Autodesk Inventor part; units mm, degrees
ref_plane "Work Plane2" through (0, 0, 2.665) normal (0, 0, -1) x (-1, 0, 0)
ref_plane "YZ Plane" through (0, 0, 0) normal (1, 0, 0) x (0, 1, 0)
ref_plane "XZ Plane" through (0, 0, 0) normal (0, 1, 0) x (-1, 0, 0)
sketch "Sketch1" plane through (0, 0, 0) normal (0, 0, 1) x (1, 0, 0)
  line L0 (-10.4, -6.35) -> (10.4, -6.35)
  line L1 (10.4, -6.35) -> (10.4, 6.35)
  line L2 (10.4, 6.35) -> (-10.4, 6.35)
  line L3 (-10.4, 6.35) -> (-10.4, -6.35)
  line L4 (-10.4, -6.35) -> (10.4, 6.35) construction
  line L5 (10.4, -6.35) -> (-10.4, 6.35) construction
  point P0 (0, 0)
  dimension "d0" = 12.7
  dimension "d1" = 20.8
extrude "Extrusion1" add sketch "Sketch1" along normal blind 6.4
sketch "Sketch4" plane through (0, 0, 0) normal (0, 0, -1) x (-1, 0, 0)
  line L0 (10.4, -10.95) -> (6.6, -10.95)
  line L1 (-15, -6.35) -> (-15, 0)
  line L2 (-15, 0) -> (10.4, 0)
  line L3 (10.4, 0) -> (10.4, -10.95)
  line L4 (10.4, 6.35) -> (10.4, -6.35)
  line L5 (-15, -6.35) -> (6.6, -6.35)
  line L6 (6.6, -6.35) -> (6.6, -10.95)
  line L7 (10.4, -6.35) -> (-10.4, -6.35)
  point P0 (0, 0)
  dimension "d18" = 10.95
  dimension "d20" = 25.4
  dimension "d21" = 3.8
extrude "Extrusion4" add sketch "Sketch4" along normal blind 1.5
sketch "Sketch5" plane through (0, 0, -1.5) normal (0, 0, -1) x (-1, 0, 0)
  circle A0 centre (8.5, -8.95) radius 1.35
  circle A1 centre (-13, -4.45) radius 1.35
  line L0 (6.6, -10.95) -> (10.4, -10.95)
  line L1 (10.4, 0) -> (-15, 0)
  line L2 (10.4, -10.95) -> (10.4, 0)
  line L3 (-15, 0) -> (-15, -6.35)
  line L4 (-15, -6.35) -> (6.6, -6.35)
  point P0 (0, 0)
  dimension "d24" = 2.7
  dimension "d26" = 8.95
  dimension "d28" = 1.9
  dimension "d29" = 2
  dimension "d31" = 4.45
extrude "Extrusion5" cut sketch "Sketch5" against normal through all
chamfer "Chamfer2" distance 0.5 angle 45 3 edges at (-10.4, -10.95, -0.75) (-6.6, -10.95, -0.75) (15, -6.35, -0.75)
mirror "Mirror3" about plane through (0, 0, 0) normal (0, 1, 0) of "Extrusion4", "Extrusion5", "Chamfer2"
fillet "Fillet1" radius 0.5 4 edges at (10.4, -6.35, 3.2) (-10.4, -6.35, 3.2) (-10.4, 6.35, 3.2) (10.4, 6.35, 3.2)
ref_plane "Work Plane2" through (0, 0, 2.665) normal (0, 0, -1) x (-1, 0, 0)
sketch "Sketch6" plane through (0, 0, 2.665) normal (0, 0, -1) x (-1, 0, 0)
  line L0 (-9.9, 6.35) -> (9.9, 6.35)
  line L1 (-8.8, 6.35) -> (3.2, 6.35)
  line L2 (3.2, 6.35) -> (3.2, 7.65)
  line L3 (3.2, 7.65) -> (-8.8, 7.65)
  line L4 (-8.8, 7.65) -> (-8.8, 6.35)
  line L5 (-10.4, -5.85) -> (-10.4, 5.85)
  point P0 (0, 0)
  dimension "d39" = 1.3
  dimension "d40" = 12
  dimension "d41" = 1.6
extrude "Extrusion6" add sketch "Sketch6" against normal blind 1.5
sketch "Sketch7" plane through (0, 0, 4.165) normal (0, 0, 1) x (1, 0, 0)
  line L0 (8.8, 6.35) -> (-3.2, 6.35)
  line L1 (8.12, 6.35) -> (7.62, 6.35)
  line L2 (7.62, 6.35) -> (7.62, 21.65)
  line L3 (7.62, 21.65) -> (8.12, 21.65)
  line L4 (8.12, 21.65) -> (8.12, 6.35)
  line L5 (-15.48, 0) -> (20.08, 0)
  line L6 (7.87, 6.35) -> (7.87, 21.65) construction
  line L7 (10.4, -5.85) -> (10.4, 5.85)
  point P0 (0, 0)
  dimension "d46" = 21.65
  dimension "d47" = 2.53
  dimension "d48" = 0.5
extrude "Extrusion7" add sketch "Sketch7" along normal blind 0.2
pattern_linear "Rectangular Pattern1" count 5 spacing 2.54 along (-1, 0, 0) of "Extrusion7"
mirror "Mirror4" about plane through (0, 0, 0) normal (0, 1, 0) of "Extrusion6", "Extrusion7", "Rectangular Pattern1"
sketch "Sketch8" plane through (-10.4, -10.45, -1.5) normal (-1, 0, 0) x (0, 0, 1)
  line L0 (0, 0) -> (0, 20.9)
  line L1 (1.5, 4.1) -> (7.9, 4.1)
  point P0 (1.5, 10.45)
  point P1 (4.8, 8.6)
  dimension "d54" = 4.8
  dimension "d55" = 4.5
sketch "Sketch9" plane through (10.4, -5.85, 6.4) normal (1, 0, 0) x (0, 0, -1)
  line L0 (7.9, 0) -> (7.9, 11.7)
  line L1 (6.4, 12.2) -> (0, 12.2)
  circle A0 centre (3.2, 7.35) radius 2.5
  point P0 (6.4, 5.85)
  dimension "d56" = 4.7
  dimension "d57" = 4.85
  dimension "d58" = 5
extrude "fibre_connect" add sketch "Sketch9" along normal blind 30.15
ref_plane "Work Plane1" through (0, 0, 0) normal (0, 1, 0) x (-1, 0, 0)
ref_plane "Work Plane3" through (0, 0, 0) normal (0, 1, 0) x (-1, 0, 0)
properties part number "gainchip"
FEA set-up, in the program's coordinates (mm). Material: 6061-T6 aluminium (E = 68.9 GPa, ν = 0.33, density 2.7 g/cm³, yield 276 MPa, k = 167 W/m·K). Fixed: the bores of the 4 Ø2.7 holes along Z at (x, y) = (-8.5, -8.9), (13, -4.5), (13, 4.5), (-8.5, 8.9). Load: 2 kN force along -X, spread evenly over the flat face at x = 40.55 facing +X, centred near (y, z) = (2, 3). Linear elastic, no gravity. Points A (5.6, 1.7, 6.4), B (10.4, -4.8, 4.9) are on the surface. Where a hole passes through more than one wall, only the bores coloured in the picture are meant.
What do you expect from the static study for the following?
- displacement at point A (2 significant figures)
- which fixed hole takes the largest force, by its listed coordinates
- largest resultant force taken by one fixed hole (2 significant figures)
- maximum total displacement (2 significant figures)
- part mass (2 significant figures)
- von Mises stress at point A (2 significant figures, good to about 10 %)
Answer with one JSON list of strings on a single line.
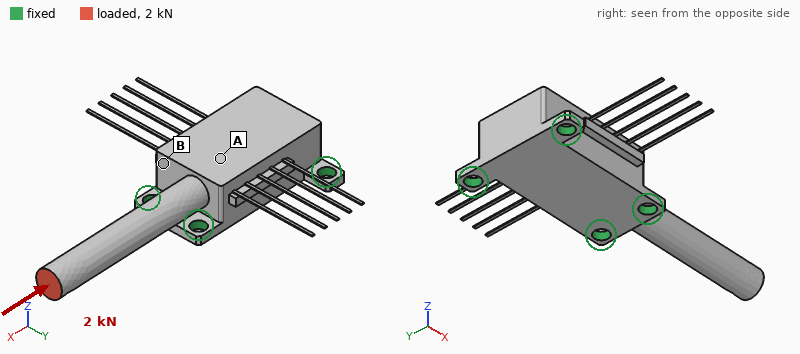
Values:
["12 µm", "(13, 4.5)", "840 N", "75 µm", "7.7 g", "50 MPa"]
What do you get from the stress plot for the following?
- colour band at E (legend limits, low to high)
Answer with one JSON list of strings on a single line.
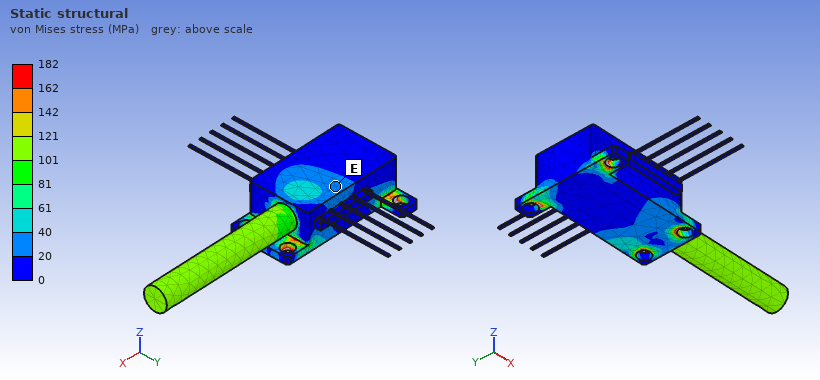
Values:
["20 to 40 MPa"]
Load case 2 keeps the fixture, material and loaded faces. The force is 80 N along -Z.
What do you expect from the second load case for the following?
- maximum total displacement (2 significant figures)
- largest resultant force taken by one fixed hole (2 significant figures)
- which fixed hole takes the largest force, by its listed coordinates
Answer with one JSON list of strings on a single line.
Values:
["0.41 mm", "120 N", "(13, 4.5)"]
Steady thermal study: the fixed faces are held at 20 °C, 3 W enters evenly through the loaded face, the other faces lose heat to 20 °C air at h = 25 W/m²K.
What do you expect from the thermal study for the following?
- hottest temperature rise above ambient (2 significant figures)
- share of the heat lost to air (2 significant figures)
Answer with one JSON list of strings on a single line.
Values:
["30 K", "8.3 %"]
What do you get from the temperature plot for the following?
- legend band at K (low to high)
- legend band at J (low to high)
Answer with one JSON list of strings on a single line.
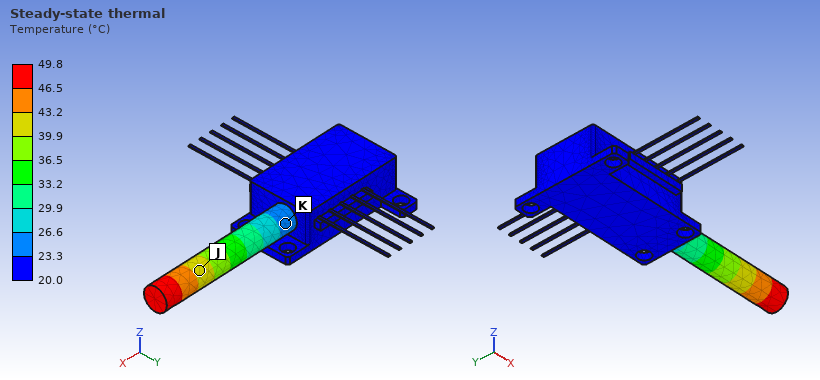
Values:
["23.3 to 26.6 °C", "39.9 to 43.2 °C"]
